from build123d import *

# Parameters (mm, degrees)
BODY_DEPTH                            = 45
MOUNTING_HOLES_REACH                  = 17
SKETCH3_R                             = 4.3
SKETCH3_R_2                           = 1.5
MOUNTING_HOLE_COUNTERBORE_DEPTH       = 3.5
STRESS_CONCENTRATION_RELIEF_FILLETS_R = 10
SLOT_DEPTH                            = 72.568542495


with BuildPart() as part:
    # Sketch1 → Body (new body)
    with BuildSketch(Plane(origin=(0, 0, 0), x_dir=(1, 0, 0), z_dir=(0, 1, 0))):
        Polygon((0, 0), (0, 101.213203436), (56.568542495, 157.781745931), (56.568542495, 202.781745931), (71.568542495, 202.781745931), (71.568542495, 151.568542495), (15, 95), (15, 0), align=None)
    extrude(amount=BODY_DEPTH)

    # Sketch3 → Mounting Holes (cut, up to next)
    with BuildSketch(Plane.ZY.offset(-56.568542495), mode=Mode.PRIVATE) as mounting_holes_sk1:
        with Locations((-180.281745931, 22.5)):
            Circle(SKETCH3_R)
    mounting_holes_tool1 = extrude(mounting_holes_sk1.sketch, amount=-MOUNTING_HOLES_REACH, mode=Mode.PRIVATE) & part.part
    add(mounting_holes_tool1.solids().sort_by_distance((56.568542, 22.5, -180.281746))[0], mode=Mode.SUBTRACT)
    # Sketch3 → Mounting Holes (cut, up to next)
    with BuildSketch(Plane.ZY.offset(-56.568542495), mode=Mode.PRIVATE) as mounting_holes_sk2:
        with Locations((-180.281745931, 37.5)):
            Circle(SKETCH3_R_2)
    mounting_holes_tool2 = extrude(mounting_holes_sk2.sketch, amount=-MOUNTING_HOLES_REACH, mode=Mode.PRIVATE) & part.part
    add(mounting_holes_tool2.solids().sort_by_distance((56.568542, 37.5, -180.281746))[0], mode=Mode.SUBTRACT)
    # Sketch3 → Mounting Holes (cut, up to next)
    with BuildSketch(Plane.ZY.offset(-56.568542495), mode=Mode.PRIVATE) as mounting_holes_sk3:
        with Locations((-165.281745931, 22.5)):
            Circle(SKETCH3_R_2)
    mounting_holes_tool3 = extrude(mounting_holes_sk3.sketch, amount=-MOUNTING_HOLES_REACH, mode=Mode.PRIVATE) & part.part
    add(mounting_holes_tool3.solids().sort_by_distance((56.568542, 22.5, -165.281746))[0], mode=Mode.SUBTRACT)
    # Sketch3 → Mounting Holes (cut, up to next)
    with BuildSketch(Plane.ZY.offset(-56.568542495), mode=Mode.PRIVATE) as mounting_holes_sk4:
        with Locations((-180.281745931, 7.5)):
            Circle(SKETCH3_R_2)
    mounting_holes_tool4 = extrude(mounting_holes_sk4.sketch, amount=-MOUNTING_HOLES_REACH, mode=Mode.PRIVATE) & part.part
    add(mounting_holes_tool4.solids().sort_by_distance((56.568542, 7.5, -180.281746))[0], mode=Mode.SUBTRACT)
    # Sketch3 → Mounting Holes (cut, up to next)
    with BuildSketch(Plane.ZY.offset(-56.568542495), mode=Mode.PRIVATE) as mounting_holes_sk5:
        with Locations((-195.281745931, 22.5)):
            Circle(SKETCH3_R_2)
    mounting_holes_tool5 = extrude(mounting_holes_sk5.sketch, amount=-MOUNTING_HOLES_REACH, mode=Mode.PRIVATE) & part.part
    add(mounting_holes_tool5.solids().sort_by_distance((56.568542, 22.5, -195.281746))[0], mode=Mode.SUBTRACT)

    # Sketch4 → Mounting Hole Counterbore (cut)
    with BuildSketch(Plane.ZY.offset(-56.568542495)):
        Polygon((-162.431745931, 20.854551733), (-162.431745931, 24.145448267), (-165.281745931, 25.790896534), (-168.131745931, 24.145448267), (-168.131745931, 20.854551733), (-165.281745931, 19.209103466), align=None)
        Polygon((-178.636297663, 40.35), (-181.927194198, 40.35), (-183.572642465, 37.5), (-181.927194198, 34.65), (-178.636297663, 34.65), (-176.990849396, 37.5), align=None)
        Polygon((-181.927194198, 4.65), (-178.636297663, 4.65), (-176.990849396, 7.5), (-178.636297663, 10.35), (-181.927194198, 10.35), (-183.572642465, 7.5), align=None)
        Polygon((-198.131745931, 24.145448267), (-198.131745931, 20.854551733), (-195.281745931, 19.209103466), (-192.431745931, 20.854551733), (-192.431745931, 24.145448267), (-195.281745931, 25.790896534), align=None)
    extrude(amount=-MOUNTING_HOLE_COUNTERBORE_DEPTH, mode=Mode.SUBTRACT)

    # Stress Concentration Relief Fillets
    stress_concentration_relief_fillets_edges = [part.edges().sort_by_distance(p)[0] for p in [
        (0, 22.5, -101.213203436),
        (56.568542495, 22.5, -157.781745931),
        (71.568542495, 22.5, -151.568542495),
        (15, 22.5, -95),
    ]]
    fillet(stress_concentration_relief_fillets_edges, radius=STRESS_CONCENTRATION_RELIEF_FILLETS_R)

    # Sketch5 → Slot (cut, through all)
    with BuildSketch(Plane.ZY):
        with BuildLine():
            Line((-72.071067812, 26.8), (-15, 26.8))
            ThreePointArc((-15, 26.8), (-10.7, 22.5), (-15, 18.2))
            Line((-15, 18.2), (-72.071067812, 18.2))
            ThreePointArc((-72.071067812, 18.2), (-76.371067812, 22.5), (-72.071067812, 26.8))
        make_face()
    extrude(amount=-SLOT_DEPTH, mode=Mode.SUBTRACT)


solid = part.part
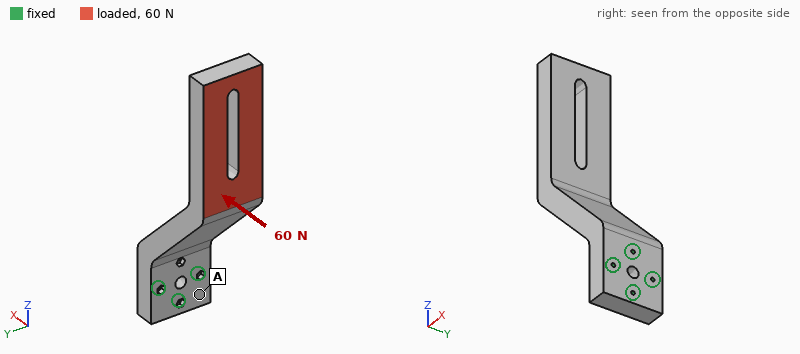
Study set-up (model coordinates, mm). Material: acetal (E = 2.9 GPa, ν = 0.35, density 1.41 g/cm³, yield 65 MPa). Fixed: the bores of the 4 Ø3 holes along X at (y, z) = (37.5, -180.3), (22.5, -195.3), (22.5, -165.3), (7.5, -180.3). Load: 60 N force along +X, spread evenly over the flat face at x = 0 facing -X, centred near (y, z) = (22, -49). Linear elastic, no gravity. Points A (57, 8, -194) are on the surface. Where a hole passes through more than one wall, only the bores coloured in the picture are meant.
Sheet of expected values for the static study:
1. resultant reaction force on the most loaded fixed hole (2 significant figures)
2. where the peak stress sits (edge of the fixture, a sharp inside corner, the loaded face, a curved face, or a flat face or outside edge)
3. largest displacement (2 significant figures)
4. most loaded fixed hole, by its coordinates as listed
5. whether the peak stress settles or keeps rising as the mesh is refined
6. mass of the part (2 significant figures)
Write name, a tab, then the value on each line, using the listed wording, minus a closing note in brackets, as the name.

resultant reaction force on the most loaded fixed hole	280 N
where the peak stress sits	edge of the fixture
largest displacement	2.1 mm
most loaded fixed hole, by its coordinates as listed	(22.5, -165.3)
whether the peak stress settles or keeps rising as the mesh is refined	keeps rising
mass of the part	200 g
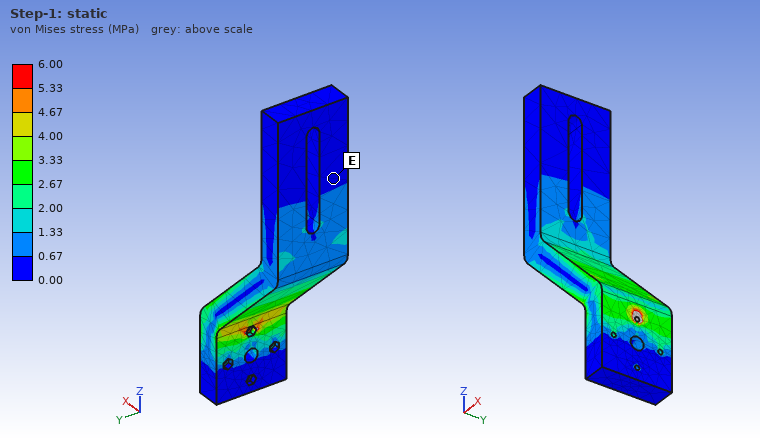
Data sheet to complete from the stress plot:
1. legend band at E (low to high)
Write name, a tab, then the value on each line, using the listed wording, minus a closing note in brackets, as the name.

legend band at E	0.00 to 0.67 MPa
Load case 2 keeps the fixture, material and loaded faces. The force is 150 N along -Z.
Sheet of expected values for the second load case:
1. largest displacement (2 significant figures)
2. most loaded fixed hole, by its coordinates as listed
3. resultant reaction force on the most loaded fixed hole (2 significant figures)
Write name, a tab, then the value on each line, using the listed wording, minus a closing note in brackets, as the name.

largest displacement	2.5 mm
most loaded fixed hole, by its coordinates as listed	(22.5, -165.3)
resultant reaction force on the most loaded fixed hole	330 N
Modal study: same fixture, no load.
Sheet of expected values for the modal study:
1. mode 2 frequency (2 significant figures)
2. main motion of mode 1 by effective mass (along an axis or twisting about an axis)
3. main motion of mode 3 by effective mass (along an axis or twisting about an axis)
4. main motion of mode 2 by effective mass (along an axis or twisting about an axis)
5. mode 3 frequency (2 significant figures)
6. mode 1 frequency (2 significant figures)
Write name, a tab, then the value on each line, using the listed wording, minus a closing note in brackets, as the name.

mode 2 frequency	220 Hz
main motion of mode 1 by effective mass	along X
main motion of mode 3 by effective mass	along Z
main motion of mode 2 by effective mass	along Y
mode 3 frequency	480 Hz
mode 1 frequency	100 Hz
